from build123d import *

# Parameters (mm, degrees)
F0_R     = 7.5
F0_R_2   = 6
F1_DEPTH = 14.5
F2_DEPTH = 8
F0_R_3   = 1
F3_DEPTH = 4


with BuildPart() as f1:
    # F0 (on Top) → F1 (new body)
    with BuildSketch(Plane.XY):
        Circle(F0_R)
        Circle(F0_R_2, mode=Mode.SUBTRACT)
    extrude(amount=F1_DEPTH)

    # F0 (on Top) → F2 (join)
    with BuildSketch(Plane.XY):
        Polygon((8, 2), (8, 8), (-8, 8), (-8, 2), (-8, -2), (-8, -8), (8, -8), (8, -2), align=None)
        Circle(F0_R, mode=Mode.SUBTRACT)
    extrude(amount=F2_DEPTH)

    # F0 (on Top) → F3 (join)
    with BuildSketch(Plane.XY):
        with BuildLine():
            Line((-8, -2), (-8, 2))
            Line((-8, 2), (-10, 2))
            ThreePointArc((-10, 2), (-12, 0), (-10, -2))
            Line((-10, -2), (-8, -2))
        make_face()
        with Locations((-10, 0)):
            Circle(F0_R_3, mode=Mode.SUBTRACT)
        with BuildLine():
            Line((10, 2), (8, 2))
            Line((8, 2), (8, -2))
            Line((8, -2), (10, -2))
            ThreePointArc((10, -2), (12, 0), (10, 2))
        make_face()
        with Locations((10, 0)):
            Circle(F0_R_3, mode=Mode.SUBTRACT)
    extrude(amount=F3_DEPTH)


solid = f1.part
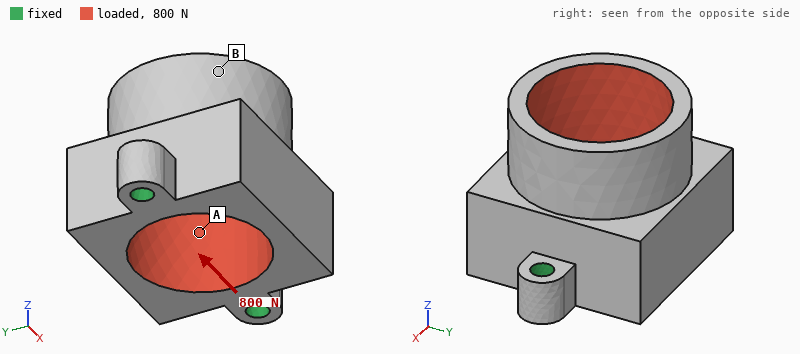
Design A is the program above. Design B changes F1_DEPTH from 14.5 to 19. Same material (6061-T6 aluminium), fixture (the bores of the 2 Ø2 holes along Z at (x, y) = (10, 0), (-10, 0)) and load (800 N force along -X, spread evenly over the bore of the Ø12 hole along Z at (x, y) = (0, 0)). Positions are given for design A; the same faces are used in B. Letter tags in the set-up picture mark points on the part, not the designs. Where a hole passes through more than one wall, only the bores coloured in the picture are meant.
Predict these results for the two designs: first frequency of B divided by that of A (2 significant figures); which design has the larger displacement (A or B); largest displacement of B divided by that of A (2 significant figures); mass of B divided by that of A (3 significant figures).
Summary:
0.75
B
1.6
1.17
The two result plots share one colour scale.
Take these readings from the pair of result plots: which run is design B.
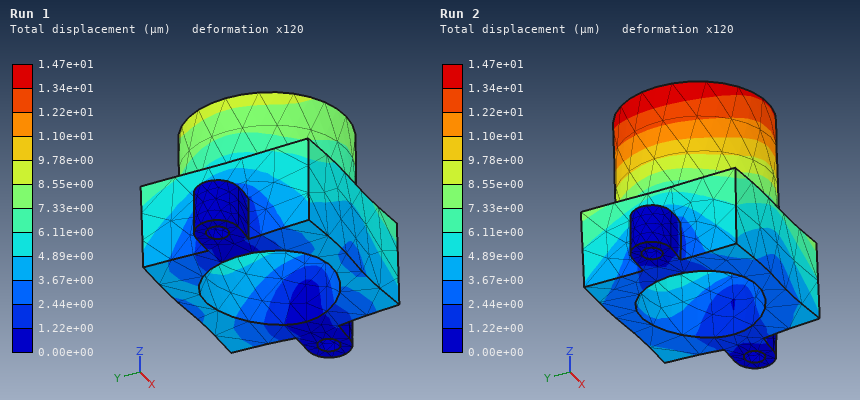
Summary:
Run 2
